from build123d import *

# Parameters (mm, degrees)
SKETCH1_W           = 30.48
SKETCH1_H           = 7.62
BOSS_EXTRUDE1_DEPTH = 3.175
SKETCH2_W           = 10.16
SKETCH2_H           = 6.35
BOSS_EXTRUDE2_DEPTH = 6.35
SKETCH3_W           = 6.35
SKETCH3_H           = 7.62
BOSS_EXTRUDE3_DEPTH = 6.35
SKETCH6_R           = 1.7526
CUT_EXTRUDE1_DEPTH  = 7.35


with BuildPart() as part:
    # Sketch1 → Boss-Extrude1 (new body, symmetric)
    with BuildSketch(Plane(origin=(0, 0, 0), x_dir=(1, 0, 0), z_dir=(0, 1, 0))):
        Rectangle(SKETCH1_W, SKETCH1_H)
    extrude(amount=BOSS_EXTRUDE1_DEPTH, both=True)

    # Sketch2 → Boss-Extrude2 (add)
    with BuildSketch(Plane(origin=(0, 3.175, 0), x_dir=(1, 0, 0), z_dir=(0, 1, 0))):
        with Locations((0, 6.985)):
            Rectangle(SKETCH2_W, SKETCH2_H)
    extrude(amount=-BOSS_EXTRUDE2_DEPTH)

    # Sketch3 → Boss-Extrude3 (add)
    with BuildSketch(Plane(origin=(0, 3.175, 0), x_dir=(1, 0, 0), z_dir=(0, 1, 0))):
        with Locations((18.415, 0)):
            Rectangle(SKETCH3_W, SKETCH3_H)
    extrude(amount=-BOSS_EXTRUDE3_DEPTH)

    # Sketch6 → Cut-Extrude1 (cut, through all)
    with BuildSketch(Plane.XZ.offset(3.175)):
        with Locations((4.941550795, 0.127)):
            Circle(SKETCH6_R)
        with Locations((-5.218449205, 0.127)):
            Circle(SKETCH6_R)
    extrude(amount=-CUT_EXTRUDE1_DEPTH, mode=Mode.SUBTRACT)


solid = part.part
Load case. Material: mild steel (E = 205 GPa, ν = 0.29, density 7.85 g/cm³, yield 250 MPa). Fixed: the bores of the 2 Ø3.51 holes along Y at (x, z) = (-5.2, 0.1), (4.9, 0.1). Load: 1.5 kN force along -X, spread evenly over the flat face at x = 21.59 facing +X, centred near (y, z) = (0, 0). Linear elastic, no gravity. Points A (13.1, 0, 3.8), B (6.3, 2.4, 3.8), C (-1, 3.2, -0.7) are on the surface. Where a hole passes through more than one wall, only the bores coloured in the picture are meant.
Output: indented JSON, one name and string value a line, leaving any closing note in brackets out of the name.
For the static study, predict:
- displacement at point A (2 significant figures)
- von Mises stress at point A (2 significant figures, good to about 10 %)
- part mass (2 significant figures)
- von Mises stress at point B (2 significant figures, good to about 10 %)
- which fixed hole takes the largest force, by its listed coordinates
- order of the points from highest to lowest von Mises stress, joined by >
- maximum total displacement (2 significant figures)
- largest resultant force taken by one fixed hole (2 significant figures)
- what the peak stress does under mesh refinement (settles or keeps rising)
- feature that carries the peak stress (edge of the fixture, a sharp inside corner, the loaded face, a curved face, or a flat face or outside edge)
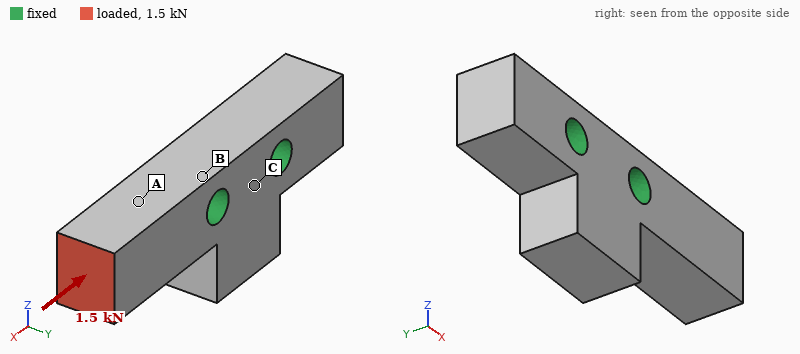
{
  "displacement at point A": "1.1 µm",
  "von Mises stress at point A": "31 MPa",
  "part mass": "16 g",
  "von Mises stress at point B": "16 MPa",
  "which fixed hole takes the largest force, by its listed coordinates": "(4.9, 0.1)",
  "order of the points from highest to lowest von Mises stress, joined by >": "A > B > C",
  "maximum total displacement": "2.5 µm",
  "largest resultant force taken by one fixed hole": "1.4 kN",
  "what the peak stress does under mesh refinement": "keeps rising",
  "feature that carries the peak stress": "edge of the fixture"
}
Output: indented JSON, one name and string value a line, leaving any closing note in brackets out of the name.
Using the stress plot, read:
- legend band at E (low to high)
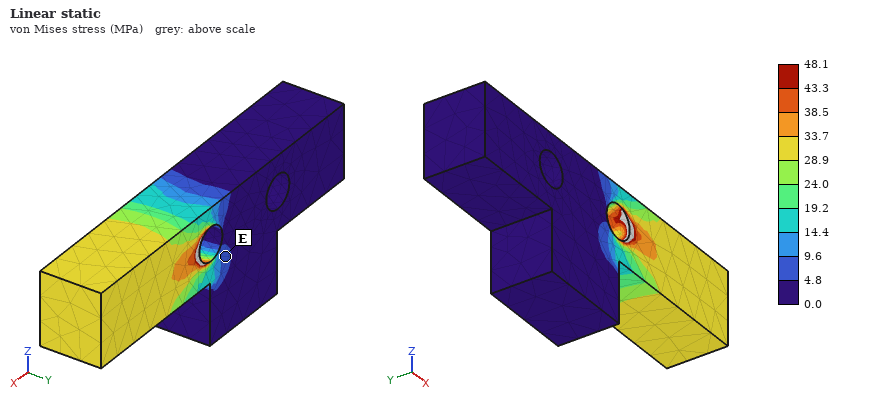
{
  "legend band at E": "4.8 to 9.6 MPa"
}
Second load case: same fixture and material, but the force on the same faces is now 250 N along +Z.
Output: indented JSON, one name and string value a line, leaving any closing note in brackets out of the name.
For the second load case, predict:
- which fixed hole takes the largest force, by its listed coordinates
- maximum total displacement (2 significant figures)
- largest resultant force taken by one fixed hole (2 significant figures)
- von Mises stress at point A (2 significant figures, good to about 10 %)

{
  "which fixed hole takes the largest force, by its listed coordinates": "(4.9, 0.1)",
  "maximum total displacement": "10 µm",
  "largest resultant force taken by one fixed hole": "360 N",
  "von Mises stress at point A": "35 MPa"
}
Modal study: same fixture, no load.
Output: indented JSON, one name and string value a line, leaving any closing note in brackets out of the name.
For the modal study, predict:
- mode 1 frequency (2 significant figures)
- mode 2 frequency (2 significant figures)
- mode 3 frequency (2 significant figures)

{
  "mode 1 frequency": "19 kHz",
  "mode 2 frequency": "19 kHz",
  "mode 3 frequency": "45 kHz"
}
